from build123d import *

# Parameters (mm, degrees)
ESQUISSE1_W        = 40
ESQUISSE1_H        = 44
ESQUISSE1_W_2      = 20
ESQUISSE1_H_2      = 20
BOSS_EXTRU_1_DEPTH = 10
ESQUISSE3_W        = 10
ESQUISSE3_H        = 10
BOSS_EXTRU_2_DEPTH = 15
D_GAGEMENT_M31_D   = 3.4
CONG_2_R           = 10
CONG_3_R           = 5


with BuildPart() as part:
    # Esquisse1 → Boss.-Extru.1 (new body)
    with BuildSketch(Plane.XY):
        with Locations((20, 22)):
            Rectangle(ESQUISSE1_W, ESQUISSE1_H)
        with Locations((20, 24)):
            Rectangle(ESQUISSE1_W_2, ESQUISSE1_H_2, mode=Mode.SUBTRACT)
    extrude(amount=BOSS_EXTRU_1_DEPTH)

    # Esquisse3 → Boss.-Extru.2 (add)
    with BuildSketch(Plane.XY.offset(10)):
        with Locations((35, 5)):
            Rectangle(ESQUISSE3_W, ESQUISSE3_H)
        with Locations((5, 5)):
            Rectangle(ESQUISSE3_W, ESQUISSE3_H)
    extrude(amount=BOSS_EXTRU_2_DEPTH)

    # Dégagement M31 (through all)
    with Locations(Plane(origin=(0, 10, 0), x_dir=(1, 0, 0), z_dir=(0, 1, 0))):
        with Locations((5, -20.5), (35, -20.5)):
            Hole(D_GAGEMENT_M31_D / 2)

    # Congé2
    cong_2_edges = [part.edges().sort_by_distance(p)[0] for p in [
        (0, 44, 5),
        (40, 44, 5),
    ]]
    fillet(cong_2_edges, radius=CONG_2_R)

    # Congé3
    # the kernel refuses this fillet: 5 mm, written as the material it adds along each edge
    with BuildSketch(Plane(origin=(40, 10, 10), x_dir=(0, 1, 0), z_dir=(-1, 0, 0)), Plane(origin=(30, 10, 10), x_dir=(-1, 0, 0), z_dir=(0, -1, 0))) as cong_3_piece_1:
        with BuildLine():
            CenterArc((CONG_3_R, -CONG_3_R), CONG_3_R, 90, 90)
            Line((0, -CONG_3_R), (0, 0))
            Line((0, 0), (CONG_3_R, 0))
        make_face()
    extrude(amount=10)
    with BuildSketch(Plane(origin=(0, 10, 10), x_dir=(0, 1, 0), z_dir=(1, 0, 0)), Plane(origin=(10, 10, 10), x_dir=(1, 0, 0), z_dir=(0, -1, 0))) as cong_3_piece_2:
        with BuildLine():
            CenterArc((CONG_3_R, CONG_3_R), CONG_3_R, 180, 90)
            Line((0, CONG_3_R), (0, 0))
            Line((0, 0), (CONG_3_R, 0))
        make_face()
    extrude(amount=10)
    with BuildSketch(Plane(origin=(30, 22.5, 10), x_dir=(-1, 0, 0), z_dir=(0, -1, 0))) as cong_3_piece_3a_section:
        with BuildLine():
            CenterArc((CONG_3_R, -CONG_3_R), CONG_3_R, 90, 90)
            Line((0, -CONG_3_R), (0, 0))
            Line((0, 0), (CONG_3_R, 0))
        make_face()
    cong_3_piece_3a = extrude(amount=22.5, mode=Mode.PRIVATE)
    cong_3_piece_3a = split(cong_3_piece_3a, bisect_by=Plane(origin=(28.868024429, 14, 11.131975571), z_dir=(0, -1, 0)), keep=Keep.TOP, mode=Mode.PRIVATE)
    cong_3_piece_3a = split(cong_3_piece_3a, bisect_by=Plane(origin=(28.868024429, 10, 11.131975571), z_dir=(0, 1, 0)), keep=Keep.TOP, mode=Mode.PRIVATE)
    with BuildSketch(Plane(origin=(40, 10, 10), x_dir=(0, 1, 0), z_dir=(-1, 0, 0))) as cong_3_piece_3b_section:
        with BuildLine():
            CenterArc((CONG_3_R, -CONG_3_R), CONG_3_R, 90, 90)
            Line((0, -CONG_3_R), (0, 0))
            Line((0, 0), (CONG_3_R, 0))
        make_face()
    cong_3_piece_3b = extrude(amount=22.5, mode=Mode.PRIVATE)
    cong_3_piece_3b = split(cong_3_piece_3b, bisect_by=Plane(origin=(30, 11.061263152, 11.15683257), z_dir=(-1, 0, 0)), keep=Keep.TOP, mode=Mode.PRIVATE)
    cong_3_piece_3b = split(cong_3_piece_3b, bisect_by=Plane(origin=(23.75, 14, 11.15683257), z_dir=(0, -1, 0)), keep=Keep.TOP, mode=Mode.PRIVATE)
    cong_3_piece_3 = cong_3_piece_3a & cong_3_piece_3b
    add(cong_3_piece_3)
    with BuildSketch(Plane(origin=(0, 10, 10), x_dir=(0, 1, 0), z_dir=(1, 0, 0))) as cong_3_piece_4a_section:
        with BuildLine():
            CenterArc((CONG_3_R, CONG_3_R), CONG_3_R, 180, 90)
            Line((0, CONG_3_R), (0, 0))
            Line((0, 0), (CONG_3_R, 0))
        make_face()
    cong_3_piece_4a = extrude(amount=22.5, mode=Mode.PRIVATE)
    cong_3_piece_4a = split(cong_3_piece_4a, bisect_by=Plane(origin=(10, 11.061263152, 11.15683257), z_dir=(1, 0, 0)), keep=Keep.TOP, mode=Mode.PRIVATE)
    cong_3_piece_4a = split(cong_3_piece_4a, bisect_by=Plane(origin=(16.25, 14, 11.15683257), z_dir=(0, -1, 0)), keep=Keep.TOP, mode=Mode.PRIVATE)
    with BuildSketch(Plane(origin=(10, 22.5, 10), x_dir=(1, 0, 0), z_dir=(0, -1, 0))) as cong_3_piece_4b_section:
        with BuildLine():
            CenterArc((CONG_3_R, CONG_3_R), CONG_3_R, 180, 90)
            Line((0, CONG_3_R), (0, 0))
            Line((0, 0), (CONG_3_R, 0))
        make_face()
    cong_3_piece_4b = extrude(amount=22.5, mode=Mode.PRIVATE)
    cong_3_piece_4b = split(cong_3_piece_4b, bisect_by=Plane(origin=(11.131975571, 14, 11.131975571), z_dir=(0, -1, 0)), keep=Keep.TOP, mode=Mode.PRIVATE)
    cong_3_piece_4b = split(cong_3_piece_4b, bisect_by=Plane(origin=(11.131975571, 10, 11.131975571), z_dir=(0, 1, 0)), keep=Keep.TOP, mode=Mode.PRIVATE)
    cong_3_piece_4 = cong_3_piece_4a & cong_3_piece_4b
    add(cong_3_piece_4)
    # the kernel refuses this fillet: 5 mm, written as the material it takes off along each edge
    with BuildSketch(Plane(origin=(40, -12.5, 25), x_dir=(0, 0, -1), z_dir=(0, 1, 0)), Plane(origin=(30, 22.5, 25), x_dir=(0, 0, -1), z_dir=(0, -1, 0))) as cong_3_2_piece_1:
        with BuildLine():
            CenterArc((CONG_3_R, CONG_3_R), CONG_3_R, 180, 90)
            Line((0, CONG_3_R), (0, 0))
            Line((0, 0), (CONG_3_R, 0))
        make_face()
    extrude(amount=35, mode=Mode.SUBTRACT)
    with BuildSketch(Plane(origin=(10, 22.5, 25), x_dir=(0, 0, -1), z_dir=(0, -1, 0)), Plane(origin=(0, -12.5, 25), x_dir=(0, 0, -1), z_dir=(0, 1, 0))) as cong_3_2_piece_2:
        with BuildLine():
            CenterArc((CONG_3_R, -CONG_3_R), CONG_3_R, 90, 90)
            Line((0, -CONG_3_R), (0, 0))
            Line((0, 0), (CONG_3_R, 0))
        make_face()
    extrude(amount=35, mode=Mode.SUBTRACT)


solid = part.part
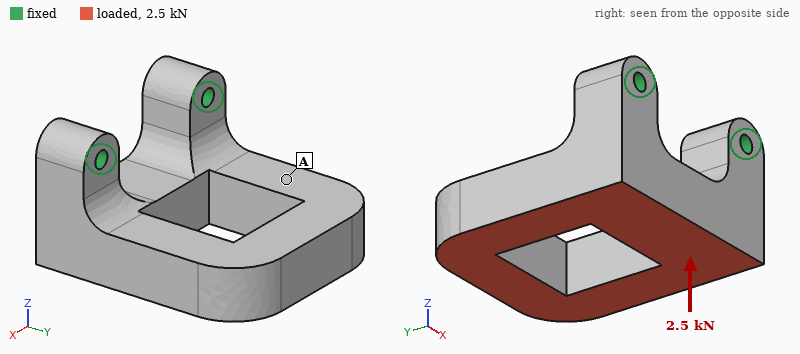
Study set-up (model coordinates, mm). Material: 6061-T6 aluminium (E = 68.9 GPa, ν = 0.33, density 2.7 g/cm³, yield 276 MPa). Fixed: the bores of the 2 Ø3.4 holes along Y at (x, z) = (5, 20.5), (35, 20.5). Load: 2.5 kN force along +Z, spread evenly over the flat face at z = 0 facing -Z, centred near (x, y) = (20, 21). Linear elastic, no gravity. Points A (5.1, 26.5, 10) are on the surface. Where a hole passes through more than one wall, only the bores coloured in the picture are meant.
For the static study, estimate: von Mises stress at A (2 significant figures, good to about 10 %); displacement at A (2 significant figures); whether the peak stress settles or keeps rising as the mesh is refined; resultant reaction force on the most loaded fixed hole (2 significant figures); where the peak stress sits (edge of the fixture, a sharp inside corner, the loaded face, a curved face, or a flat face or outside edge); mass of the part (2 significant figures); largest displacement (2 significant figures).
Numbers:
27 MPa
0.12 mm
keeps rising
1.3 kN
edge of the fixture
43 g
0.26 mm
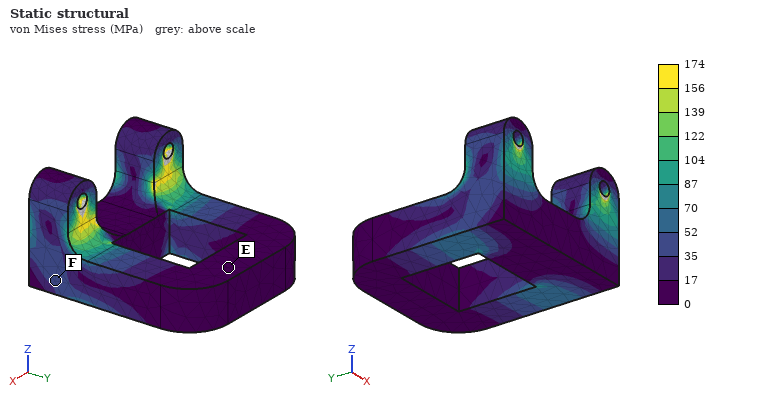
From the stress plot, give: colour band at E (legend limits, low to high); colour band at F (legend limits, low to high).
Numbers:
0 to 17 MPa
35 to 52 MPa
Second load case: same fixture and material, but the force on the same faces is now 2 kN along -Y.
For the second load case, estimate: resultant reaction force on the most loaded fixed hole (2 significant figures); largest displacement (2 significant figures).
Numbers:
1.0 kN
0.16 mm
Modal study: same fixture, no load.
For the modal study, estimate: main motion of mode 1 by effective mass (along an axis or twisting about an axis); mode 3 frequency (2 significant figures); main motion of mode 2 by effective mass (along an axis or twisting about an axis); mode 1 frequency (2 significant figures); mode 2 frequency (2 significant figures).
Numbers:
along Z
8800 Hz
along X
3100 Hz
5100 Hz
